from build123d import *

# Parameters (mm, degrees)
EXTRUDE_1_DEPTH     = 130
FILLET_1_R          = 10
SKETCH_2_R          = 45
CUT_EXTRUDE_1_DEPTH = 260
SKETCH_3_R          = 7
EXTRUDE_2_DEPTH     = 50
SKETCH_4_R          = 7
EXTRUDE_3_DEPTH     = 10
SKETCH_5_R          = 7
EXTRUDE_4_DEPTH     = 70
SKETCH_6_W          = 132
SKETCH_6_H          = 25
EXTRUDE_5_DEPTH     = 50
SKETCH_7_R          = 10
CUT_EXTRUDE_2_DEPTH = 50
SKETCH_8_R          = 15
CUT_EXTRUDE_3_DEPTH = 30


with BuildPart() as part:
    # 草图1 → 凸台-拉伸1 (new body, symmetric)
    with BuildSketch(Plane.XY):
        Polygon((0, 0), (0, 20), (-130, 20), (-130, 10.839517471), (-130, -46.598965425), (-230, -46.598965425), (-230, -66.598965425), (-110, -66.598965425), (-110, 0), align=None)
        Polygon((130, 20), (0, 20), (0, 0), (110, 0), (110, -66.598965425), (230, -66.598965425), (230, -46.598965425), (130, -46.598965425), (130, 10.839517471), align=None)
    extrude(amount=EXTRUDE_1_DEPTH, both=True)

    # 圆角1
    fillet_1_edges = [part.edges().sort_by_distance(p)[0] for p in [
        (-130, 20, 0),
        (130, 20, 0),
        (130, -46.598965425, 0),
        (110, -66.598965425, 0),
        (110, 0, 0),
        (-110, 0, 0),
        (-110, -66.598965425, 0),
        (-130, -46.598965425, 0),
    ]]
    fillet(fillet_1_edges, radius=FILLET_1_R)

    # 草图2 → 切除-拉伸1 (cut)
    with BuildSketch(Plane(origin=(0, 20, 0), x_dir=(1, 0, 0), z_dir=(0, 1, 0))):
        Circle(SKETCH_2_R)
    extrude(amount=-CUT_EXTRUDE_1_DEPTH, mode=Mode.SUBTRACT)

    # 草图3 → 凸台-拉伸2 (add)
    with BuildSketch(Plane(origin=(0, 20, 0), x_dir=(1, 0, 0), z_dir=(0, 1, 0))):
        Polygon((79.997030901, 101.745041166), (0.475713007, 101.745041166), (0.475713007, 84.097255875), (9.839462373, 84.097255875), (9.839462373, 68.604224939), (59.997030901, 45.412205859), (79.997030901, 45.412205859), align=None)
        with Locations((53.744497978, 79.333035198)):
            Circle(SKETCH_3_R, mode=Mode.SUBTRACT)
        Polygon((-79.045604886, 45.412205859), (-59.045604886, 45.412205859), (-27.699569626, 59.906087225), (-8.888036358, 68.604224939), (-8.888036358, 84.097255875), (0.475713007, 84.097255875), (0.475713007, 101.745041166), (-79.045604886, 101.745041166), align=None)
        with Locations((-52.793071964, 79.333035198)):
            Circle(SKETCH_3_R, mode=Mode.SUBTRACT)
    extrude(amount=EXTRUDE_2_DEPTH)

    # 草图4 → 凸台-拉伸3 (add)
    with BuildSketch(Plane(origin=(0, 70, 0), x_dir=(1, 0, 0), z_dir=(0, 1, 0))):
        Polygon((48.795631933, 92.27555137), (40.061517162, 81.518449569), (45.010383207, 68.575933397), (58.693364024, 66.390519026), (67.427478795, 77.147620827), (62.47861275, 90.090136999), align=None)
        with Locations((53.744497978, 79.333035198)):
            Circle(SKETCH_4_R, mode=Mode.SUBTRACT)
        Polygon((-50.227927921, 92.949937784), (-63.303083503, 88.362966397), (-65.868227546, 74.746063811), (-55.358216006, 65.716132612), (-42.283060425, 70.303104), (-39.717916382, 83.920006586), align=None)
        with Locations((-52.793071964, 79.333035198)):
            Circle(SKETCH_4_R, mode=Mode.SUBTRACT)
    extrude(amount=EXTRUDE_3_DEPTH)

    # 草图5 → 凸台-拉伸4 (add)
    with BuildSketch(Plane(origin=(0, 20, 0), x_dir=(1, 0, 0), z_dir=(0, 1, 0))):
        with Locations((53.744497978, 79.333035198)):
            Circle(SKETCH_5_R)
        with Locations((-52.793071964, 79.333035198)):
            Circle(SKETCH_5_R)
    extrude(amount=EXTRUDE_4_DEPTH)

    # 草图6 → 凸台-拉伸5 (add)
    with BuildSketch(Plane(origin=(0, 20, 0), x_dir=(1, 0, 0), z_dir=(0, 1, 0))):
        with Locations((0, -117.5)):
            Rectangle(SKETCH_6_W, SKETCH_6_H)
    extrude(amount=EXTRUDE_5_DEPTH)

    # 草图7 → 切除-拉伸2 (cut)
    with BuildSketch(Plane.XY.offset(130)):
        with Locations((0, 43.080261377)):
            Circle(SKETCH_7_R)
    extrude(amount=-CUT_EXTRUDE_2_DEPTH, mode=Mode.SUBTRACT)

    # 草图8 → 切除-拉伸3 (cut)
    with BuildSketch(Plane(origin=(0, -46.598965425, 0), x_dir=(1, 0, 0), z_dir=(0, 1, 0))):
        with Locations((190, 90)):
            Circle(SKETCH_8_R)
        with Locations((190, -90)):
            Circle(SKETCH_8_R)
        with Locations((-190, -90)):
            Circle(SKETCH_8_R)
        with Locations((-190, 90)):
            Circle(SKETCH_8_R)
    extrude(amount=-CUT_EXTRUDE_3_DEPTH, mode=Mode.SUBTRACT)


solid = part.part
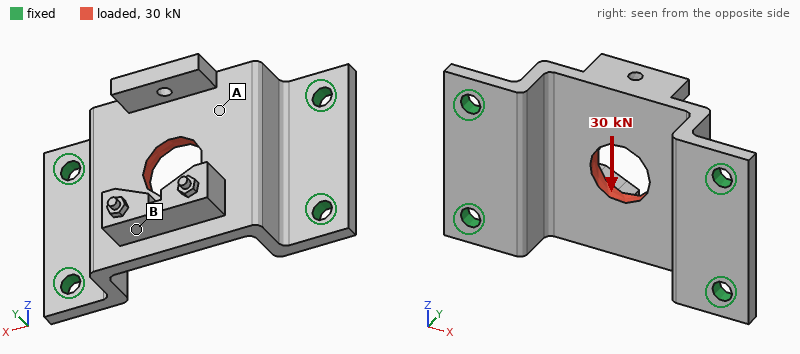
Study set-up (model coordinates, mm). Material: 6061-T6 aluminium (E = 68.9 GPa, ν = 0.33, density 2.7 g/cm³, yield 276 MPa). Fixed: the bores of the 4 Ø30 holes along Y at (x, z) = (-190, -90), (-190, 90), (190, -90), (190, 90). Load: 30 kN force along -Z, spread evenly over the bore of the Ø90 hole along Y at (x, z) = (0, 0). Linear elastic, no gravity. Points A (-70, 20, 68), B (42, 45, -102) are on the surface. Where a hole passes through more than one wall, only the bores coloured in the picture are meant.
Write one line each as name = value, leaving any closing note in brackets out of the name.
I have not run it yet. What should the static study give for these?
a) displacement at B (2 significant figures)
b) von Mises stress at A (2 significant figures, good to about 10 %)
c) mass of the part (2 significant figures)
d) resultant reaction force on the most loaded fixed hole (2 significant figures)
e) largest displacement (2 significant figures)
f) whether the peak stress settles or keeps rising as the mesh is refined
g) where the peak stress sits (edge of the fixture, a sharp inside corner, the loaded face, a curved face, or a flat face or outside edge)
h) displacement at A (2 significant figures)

displacement at B = 72 µm
von Mises stress at A = 5.6 MPa
mass of the part = 9.2 kg
resultant reaction force on the most loaded fixed hole = 12 kN
largest displacement = 92 µm
whether the peak stress settles or keeps rising as the mesh is refined = keeps rising
where the peak stress sits = edge of the fixture
displacement at A = 57 µm
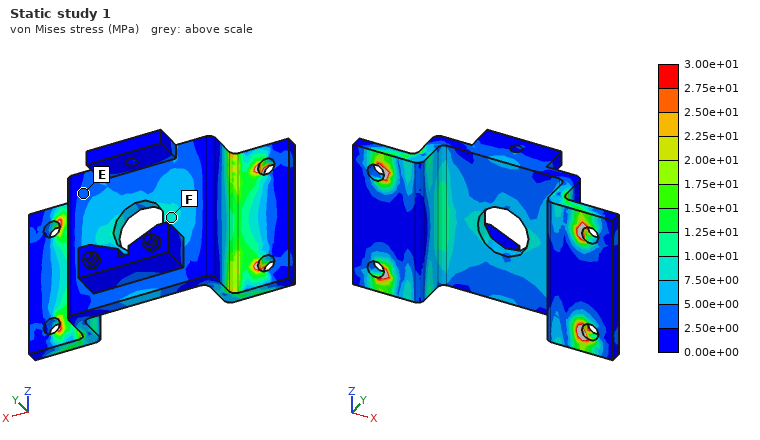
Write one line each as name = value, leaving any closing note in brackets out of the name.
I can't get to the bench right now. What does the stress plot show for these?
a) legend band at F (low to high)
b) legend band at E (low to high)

legend band at F = 7.50e+00 to 1.00e+01 MPa
legend band at E = 2.50e+00 to 5.00e+00 MPa
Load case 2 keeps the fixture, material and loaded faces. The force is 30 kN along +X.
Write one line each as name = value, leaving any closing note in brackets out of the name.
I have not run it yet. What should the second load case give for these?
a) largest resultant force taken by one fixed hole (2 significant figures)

largest resultant force taken by one fixed hole = 8.2 kN
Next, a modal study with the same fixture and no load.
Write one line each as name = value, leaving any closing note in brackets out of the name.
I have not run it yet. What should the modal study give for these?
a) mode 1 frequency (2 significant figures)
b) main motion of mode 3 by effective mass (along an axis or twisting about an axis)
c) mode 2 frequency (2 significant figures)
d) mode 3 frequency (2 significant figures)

mode 1 frequency = 1100 Hz
main motion of mode 3 by effective mass = along Y
mode 2 frequency = 1200 Hz
mode 3 frequency = 1300 Hz
